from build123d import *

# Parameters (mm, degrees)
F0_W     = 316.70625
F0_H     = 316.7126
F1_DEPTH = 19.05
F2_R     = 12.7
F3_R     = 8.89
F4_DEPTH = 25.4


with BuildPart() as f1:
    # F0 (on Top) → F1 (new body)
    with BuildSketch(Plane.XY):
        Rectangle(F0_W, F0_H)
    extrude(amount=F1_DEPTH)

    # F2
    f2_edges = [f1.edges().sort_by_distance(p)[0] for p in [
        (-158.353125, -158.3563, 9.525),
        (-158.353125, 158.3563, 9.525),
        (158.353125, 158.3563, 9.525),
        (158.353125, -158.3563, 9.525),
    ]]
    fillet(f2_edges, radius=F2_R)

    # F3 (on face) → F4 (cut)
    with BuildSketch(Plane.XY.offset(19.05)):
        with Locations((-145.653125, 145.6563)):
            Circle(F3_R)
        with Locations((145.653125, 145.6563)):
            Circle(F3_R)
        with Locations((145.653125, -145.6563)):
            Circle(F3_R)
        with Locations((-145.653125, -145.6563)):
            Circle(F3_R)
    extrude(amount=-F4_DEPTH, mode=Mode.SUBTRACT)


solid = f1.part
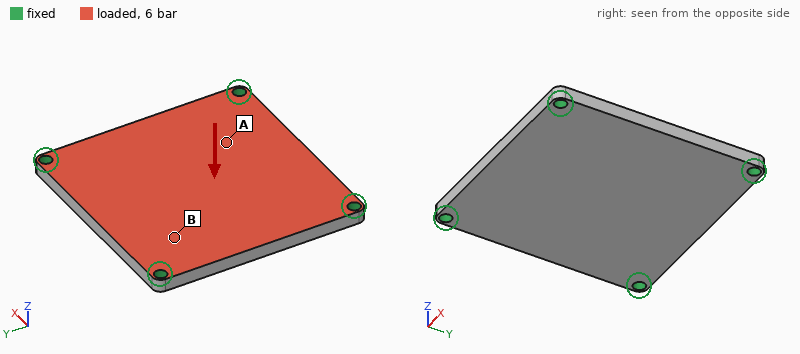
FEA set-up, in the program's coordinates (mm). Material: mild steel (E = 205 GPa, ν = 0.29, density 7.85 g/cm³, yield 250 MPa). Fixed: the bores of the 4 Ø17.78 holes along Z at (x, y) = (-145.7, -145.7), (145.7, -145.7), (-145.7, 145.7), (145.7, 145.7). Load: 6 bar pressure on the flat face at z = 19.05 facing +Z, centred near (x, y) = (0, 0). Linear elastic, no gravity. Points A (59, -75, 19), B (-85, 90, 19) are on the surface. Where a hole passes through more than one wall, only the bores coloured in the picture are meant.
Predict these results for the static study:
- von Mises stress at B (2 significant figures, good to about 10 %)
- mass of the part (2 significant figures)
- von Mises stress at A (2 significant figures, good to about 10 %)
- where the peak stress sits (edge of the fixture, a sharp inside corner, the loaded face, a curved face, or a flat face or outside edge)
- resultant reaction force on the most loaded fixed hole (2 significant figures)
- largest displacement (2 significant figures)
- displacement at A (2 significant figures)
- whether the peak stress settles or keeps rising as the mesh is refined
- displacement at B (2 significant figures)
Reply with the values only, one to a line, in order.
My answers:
22 MPa
15 kg
35 MPa
edge of the fixture
15 kN
0.30 mm
0.21 mm
keeps rising
0.16 mm
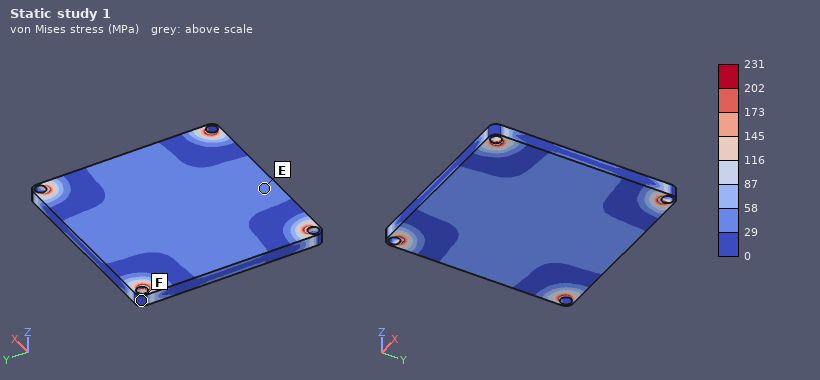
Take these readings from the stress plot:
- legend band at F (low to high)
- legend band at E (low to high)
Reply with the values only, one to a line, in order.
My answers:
0 to 29 MPa
29 to 58 MPa
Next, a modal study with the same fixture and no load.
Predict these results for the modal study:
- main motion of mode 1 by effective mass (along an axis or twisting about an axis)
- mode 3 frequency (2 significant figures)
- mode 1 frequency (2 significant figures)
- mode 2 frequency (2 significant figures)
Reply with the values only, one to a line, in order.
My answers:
along Z
1300 Hz
700 Hz
1300 Hz
